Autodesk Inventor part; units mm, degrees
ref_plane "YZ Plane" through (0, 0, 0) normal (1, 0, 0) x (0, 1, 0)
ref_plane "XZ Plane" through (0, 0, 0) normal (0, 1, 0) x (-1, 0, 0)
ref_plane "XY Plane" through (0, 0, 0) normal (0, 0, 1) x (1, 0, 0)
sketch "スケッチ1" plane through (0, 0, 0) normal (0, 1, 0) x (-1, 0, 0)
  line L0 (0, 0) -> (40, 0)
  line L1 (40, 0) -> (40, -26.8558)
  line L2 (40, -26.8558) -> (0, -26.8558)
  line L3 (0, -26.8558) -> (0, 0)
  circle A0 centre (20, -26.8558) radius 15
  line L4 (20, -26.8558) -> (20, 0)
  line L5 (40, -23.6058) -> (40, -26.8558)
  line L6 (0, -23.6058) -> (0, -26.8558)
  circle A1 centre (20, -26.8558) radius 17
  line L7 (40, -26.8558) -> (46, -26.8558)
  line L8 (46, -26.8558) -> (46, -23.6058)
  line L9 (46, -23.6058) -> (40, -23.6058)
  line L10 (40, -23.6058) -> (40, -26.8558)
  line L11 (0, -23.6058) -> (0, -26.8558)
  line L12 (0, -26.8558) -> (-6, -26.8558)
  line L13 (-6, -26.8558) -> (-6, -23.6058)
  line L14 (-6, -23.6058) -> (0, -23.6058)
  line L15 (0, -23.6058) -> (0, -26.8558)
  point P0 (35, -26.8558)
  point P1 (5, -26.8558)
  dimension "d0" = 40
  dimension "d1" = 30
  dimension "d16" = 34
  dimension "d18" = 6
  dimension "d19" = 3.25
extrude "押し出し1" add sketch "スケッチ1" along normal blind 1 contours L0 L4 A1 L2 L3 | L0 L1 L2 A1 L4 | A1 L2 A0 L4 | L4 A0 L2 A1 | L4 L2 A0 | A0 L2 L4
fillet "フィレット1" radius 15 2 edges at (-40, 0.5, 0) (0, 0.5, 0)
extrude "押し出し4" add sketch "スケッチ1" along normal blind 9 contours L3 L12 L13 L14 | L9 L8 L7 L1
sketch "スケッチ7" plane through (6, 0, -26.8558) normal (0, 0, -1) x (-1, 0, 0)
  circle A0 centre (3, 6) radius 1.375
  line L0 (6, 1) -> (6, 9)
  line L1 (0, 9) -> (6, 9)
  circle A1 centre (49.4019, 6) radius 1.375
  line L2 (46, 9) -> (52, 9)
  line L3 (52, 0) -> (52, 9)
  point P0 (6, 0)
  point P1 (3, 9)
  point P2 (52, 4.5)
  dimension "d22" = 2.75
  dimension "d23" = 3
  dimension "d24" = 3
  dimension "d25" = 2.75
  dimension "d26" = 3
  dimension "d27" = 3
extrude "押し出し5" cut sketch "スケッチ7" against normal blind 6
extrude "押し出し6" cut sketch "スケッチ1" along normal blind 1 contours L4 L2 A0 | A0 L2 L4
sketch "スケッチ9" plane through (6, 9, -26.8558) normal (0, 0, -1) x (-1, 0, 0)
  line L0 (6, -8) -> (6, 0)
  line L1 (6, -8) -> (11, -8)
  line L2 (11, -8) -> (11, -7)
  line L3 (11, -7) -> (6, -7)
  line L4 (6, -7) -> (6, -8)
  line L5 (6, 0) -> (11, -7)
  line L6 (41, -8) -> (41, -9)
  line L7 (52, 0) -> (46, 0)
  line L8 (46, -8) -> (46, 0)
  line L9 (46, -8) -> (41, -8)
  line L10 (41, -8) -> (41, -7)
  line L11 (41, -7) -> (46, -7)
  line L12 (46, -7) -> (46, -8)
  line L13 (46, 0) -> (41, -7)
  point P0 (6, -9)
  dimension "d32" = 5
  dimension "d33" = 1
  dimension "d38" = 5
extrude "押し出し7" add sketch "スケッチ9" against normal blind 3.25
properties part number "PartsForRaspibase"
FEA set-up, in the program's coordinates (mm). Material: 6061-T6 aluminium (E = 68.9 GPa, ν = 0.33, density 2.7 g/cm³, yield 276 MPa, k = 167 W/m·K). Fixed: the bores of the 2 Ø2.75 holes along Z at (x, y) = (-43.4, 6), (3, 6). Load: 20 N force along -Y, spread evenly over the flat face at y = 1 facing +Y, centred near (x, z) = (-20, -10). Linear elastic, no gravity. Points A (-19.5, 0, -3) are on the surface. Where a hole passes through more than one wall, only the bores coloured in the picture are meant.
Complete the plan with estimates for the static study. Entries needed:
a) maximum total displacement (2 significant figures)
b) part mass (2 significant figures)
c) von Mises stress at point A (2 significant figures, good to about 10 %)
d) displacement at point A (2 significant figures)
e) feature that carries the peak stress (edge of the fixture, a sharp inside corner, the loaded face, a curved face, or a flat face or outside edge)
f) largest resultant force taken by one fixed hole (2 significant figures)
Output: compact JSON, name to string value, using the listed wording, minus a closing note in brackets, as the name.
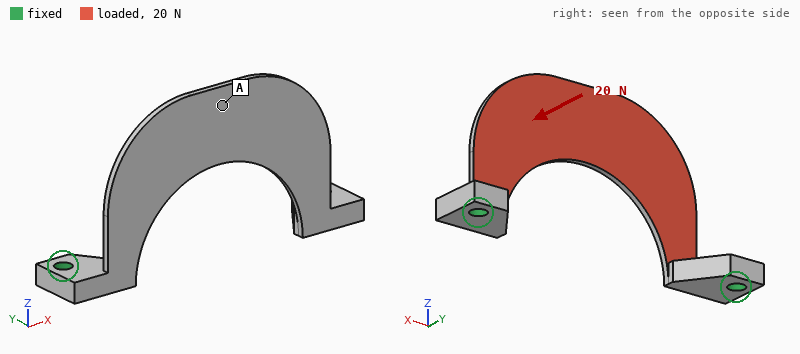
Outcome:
{"maximum total displacement": "0.62 mm", "part mass": "2.9 g", "von Mises stress at point A": "18 MPa", "displacement at point A": "0.53 mm", "feature that carries the peak stress": "a curved face", "largest resultant force taken by one fixed hole": "10 N"}
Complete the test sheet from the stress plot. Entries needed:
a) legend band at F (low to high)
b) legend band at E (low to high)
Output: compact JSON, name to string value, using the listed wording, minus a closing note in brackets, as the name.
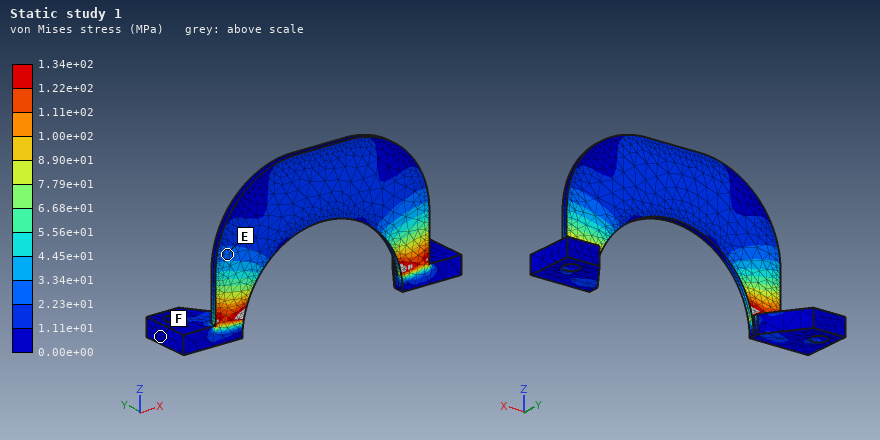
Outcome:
{"legend band at F": "0.00e+00 to 1.11e+01 MPa", "legend band at E": "2.23e+01 to 3.34e+01 MPa"}
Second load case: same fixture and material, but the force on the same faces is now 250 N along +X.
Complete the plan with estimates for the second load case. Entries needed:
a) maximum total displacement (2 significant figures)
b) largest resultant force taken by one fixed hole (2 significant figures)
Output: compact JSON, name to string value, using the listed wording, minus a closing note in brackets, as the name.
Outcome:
{"maximum total displacement": "70 µm", "largest resultant force taken by one fixed hole": "150 N"}
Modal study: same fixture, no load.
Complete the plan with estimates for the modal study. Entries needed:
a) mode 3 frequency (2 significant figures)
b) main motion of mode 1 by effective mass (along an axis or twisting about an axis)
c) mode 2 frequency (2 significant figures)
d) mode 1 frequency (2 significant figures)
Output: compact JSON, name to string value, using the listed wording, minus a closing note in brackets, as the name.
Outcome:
{"mode 3 frequency": "5800 Hz", "main motion of mode 1 by effective mass": "along Y", "mode 2 frequency": "2700 Hz", "mode 1 frequency": "900 Hz"}
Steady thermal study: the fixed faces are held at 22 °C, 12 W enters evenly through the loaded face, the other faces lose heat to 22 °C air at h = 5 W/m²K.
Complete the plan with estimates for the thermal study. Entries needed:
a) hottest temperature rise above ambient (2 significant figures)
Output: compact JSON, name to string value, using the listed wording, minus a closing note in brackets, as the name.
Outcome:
{"hottest temperature rise above ambient": "82 K"}
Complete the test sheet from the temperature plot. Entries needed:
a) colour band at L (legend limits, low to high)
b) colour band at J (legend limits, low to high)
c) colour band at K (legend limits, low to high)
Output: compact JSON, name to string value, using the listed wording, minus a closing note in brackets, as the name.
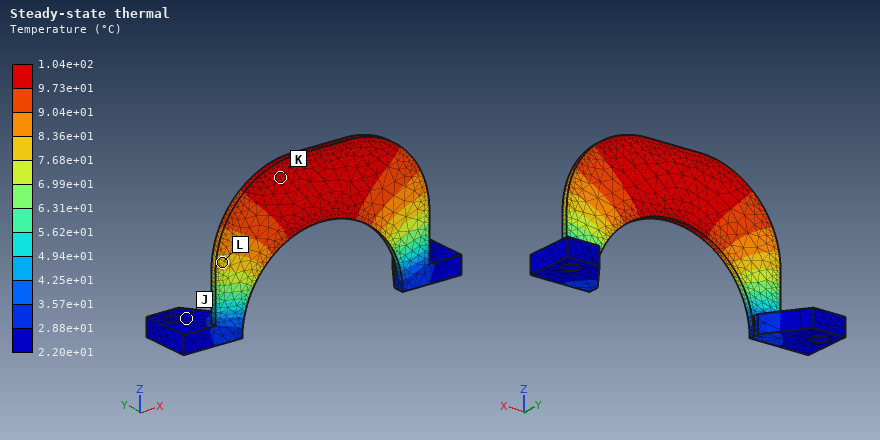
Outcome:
{"colour band at L": "7.68e+01 to 8.36e+01 °C", "colour band at J": "2.20e+01 to 2.88e+01 °C", "colour band at K": "9.73e+01 to 1.04e+02 °C"}
